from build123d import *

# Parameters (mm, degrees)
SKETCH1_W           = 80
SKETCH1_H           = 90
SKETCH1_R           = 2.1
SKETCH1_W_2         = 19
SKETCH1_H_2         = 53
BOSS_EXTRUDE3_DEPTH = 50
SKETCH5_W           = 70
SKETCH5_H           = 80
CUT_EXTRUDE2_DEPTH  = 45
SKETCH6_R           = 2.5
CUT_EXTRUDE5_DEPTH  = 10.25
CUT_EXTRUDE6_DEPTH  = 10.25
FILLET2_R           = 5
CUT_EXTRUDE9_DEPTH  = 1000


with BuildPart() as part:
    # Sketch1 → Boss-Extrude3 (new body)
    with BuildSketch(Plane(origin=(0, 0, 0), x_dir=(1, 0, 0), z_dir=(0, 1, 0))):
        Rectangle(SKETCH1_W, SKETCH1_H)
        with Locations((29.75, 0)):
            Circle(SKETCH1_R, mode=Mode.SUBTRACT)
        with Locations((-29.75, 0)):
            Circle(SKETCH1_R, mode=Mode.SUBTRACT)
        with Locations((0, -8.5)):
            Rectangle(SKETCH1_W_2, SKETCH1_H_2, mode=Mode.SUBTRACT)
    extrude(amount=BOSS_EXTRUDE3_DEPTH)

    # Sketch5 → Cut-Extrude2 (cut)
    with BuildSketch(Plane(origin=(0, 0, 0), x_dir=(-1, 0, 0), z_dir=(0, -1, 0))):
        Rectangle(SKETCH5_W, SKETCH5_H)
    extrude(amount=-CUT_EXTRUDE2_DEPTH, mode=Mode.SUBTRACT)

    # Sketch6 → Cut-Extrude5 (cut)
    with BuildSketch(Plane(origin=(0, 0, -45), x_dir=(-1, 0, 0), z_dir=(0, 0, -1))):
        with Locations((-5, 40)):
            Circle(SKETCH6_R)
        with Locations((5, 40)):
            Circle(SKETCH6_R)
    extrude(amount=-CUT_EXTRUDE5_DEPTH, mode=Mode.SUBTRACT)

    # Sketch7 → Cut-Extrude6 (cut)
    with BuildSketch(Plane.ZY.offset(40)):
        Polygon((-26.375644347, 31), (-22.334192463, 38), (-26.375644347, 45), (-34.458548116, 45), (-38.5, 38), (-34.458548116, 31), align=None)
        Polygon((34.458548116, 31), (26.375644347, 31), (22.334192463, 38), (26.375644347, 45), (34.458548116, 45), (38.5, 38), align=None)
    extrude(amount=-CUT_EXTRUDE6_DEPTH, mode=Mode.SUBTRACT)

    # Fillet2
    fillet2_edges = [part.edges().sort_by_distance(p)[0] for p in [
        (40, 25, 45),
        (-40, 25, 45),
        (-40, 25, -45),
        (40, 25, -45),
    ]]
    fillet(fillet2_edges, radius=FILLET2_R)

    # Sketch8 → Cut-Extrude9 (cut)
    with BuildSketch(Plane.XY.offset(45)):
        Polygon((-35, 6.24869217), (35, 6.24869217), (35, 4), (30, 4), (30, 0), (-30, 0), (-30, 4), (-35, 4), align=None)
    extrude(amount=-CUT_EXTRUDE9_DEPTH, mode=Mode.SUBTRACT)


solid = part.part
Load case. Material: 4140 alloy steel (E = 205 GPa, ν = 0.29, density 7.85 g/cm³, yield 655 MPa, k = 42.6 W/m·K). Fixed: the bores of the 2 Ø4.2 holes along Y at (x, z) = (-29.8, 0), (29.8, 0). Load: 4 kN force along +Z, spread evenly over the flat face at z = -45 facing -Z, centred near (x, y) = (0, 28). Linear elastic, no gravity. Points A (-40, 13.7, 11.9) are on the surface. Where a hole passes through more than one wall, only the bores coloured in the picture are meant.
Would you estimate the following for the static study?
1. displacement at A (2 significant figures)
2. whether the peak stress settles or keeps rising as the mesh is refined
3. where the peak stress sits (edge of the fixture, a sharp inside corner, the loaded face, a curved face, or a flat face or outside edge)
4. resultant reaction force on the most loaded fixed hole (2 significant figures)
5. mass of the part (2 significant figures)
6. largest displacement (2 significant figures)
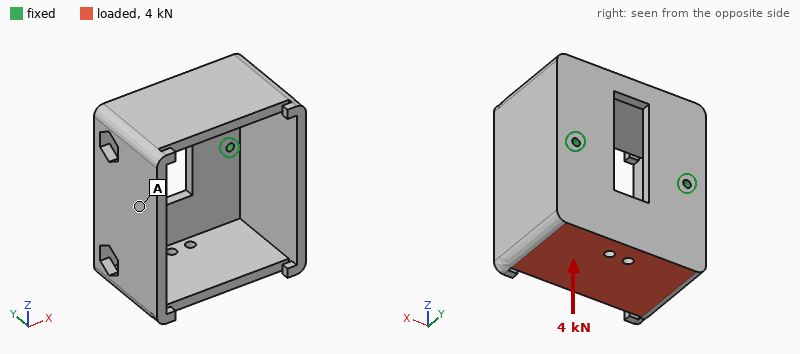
0.11 mm
keeps rising
edge of the fixture
2.0 kN
750 g
0.23 mm
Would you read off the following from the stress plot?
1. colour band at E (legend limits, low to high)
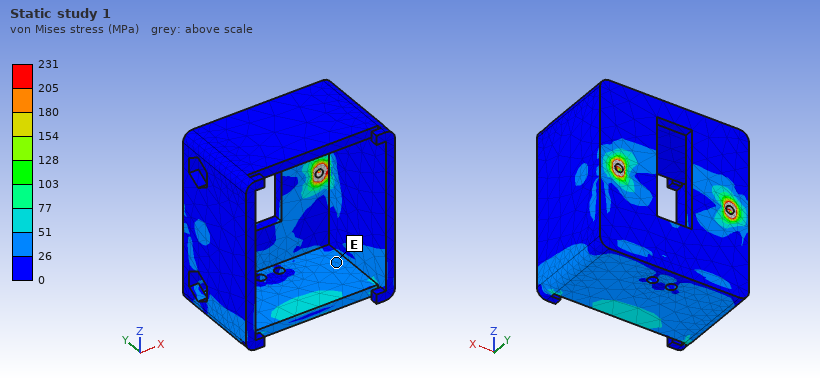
26 to 51 MPa
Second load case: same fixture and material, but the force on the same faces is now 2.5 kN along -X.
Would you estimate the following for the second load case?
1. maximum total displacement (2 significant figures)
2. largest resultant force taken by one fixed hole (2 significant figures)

58 µm
2.3 kN
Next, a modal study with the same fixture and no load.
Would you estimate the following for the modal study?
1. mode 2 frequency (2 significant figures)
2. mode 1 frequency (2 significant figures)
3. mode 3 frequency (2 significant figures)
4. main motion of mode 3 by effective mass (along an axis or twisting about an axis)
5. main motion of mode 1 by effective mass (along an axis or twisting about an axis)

1500 Hz
780 Hz
2600 Hz
along X
along Z
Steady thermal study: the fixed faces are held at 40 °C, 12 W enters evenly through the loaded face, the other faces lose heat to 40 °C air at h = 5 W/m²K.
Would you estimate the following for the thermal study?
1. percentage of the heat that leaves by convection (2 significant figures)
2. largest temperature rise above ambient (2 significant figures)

18 %
29 K
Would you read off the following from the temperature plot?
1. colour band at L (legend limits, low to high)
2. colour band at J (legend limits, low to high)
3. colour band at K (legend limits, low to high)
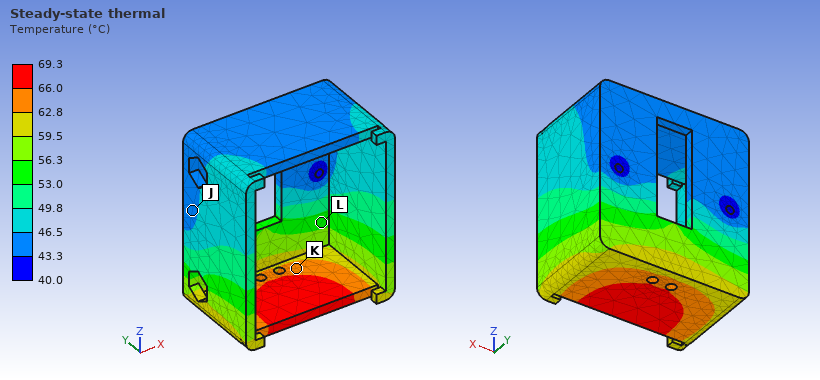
53.0 to 56.3 °C
43.3 to 46.5 °C
62.8 to 66.0 °C
